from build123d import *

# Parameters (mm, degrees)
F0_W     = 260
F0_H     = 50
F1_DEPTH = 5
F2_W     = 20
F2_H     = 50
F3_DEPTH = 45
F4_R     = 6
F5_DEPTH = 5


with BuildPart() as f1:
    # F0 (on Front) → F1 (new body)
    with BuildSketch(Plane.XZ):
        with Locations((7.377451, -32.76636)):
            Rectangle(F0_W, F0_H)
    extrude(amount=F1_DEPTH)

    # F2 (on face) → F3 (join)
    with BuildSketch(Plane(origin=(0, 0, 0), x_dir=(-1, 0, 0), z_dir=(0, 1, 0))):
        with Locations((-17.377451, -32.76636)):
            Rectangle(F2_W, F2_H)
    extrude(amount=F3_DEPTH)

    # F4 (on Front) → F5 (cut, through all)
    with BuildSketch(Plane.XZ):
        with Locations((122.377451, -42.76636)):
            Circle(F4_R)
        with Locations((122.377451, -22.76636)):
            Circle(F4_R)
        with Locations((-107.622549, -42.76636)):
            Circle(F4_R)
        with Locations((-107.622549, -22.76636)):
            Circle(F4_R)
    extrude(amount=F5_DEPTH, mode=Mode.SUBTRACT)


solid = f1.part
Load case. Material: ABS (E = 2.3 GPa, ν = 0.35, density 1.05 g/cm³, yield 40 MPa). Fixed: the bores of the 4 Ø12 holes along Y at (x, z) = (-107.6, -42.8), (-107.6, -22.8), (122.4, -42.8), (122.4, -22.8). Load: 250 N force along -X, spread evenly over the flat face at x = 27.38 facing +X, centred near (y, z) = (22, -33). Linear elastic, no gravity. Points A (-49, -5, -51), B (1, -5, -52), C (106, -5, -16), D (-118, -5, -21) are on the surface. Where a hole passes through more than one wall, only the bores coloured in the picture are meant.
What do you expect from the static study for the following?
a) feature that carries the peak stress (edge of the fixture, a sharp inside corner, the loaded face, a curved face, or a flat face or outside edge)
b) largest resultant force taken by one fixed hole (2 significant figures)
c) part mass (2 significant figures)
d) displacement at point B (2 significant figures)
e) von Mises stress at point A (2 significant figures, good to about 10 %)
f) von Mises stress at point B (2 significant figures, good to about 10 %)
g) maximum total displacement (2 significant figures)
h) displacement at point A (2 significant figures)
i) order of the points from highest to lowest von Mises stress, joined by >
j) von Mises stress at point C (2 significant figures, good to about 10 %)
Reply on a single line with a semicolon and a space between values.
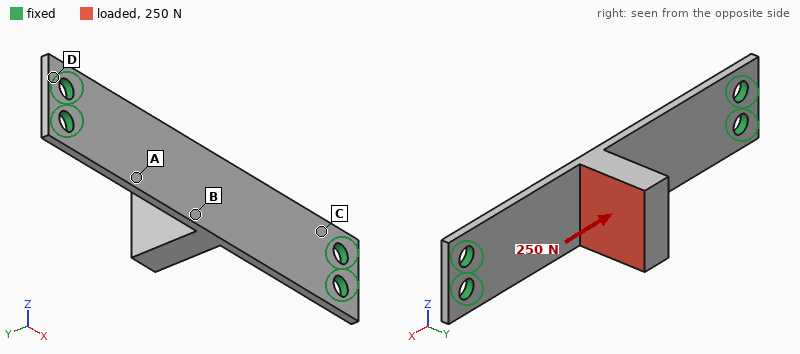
a flat face or outside edge; 71 N; 110 g; 1.4 mm; 2.2 MPa; 11 MPa; 2.8 mm; 1.2 mm; B > C > A > D; 3.8 MPa
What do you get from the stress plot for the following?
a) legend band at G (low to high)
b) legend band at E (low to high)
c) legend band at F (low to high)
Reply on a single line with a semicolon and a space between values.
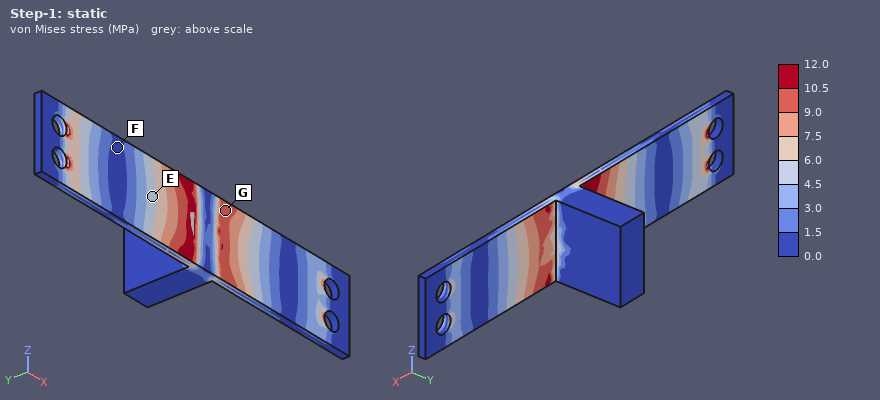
9.0 to 10.5 MPa; 4.5 to 6.0 MPa; 0.0 to 1.5 MPa
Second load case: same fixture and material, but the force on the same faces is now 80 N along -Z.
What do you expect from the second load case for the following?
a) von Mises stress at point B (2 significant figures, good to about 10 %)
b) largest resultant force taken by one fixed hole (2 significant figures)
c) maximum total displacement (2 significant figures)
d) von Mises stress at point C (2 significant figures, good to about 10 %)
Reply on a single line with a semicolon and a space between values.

3.3 MPa; 93 N; 2.7 mm; 3.6 MPa
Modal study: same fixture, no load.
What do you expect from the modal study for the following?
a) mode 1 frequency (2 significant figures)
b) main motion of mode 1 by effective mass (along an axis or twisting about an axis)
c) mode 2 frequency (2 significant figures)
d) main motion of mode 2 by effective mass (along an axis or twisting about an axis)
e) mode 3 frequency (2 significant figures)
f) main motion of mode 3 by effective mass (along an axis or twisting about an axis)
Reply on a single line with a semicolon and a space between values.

100 Hz; along Y; 140 Hz; along Z; 250 Hz; along X
